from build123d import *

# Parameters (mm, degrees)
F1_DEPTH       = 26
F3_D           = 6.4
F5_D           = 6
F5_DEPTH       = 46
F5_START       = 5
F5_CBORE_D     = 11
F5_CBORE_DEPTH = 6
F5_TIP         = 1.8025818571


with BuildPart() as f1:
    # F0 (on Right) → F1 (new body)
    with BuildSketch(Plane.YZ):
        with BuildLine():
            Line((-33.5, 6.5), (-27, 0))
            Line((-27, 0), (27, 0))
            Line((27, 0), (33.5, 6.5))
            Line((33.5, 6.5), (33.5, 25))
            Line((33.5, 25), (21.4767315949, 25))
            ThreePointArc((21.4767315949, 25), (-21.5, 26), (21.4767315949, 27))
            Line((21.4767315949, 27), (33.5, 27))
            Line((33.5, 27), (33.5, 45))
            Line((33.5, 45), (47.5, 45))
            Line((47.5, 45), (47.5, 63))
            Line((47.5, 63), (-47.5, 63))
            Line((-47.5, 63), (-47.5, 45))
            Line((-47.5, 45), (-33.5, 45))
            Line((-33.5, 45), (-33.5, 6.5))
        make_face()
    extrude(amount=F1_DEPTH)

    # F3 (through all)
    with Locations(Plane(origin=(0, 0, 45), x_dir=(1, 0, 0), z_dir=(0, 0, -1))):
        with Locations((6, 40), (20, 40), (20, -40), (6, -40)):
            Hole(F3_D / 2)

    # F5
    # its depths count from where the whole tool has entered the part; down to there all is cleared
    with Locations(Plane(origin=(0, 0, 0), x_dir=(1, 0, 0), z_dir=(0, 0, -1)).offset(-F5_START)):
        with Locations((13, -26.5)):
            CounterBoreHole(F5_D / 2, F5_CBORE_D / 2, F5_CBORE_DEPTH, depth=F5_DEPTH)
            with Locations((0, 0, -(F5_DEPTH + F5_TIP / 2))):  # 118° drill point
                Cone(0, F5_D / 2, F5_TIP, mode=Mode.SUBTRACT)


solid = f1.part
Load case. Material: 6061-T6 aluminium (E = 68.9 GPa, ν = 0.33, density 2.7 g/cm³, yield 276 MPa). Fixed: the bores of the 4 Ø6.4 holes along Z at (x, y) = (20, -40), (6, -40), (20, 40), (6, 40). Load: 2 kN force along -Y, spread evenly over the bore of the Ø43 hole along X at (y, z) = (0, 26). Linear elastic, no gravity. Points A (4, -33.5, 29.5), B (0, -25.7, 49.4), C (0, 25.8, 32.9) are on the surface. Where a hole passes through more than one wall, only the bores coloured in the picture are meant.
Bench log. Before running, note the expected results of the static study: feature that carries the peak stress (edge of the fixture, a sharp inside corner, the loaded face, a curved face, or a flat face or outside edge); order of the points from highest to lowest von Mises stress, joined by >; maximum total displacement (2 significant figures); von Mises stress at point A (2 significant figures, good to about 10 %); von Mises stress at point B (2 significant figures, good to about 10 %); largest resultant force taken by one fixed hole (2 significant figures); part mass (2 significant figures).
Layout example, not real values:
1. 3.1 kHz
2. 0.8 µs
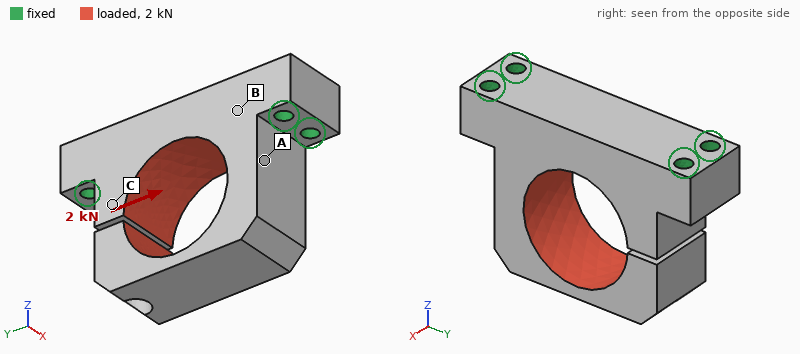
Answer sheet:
1. the loaded face
2. A > B > C
3. 0.16 mm
4. 24 MPa
5. 12 MPa
6. 810 N
7. 210 g
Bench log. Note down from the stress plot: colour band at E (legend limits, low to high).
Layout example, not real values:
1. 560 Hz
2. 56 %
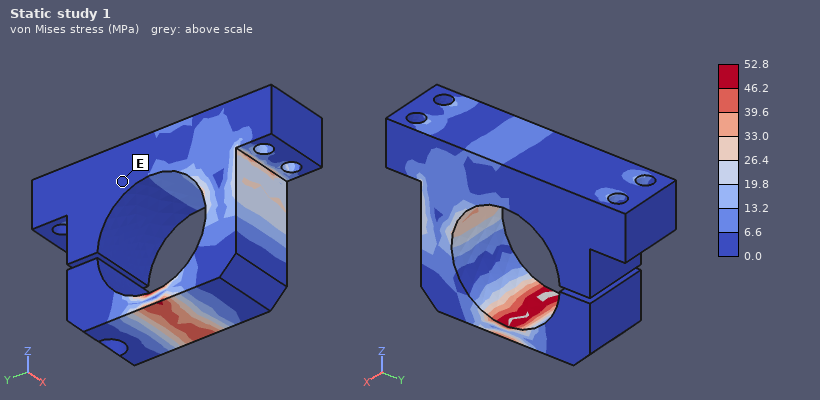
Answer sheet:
1. 0.0 to 6.6 MPa
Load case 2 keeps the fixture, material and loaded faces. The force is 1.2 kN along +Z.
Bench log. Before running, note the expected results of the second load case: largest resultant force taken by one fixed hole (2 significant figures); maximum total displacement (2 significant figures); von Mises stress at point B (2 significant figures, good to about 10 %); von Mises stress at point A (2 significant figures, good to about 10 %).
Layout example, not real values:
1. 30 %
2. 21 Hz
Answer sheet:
1. 330 N
2. 0.32 mm
3. 8.6 MPa
4. 21 MPa
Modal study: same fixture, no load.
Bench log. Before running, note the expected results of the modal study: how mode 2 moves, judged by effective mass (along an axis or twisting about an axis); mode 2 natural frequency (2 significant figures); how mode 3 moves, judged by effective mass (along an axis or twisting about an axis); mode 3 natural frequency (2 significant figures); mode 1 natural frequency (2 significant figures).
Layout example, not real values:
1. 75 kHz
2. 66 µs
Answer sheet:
1. along X
2. 1500 Hz
3. along Y
4. 2200 Hz
5. 920 Hz
